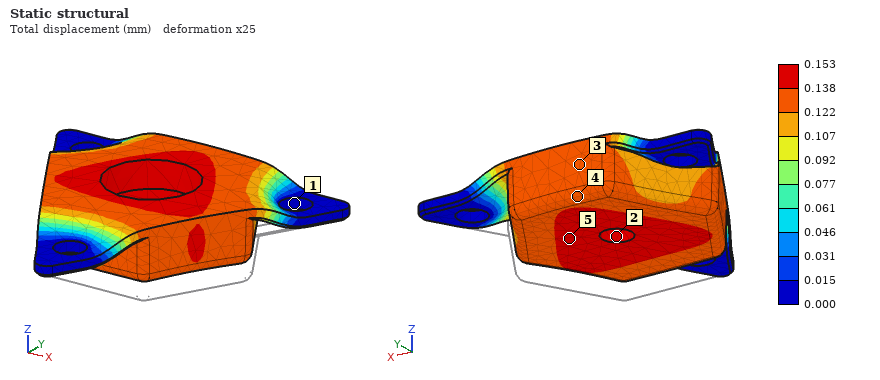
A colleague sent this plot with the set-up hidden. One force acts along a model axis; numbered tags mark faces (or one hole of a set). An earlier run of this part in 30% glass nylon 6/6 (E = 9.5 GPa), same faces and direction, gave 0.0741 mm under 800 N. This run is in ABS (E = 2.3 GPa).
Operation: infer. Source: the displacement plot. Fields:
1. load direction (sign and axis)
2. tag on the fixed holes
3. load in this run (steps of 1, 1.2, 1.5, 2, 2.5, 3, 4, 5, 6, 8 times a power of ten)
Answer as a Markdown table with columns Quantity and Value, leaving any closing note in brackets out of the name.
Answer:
| Quantity | Value |
|---|---|
| load direction | +Z |
| tag on the fixed holes | 1 |
| load in this run | 400 N |
